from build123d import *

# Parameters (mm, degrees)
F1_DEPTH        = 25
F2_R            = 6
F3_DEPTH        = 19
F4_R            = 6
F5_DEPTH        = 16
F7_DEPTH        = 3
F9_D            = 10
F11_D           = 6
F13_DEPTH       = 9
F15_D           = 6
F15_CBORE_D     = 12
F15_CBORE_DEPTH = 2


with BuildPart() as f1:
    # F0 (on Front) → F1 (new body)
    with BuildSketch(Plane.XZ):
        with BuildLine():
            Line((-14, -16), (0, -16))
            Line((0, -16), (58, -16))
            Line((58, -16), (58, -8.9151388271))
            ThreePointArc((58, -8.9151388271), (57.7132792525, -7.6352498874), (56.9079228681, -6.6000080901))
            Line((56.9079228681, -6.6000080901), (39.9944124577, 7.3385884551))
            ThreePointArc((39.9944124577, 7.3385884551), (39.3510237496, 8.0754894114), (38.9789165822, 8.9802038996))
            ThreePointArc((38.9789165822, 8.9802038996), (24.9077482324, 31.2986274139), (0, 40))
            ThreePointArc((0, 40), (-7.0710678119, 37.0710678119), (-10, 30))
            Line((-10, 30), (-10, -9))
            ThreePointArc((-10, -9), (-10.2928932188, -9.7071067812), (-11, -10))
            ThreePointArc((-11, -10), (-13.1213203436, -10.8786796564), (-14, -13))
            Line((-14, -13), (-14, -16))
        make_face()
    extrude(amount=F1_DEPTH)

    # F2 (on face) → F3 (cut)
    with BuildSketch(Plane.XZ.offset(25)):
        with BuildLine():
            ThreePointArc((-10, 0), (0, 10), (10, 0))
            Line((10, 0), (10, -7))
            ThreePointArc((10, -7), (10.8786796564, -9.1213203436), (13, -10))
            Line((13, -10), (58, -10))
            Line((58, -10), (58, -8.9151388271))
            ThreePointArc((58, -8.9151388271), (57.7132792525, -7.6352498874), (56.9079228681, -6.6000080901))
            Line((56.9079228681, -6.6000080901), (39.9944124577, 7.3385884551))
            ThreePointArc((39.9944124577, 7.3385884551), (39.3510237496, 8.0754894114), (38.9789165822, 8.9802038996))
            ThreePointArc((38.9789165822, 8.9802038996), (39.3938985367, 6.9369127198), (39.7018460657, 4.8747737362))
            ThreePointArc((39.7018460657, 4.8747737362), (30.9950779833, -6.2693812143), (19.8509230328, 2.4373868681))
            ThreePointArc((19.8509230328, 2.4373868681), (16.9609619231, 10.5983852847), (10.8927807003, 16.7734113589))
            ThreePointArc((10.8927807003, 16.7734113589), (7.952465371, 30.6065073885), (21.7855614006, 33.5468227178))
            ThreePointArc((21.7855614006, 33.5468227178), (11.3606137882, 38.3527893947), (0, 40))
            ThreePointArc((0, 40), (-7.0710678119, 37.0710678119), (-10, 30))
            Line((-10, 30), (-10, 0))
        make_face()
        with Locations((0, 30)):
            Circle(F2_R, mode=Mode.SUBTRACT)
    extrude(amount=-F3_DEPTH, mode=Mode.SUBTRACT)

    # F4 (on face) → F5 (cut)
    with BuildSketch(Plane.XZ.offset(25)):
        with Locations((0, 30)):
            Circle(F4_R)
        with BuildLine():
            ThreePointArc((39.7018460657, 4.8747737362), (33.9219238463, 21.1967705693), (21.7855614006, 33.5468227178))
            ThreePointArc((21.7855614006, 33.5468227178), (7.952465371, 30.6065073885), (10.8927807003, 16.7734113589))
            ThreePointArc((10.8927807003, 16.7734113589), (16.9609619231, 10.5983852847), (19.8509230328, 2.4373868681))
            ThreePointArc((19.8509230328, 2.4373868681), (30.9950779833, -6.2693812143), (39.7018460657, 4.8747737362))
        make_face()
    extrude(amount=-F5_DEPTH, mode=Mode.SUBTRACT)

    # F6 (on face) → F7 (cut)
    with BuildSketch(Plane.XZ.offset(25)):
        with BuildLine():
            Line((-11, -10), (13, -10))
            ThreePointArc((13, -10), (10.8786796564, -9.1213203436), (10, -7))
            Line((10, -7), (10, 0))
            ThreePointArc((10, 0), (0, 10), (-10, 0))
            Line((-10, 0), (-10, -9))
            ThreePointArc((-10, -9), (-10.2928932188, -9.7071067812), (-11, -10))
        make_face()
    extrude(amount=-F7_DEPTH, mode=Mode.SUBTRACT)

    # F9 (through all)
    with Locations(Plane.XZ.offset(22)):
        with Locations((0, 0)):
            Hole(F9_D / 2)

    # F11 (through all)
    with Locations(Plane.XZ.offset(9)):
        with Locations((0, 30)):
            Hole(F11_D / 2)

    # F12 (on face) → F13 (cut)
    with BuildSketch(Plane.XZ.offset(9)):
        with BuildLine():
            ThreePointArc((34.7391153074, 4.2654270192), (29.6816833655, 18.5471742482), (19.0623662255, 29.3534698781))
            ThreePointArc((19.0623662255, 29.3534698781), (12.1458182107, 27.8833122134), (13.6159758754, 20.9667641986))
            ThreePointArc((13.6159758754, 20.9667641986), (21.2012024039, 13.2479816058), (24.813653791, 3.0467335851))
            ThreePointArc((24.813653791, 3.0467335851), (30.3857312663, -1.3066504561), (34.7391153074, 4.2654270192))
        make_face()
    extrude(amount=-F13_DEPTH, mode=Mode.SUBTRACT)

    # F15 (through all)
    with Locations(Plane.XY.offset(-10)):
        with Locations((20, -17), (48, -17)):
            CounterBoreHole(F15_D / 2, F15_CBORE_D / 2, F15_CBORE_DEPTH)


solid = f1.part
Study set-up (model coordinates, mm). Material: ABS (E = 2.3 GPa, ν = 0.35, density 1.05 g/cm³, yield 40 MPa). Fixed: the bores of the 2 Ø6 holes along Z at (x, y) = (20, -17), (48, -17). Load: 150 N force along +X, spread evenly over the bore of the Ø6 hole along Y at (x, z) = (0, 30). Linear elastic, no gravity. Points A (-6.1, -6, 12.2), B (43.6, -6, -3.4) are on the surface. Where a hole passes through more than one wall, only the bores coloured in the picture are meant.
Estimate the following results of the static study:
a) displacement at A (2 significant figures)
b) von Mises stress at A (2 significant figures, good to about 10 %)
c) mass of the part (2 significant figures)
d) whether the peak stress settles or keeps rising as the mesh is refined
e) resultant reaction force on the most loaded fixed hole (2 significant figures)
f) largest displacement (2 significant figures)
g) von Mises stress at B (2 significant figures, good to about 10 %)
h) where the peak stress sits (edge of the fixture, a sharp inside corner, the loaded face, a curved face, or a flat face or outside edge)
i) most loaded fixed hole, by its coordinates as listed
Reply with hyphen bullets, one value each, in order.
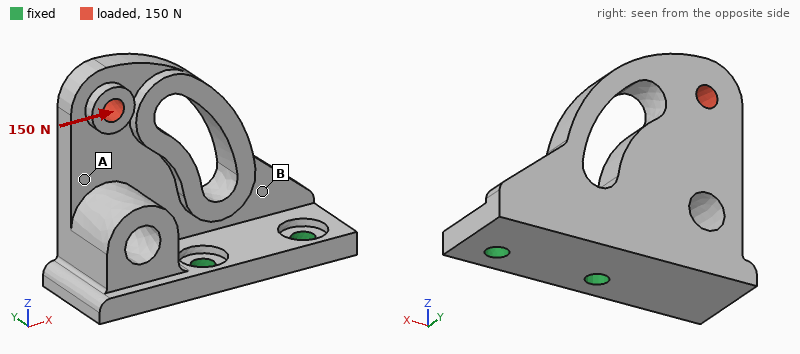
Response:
- 0.64 mm
- 2.5 MPa
- 29 g
- keeps rising
- 230 N
- 1.00 mm
- 7.3 MPa
- edge of the fixture
- (48, -17)
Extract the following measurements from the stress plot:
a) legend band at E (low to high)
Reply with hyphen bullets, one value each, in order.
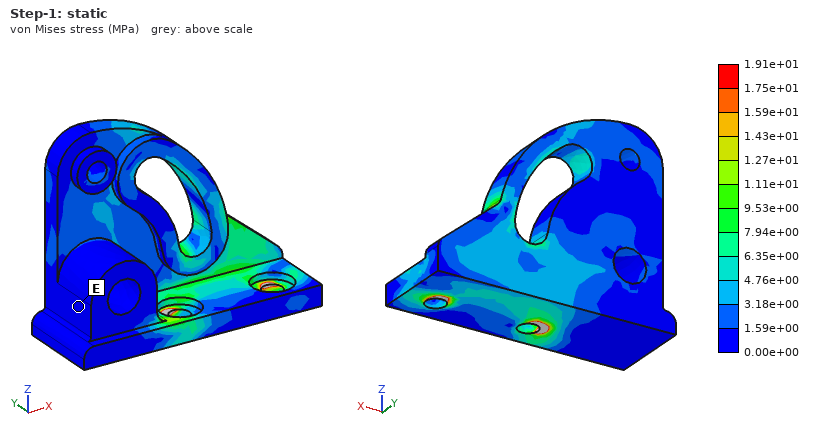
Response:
- 0.00e+00 to 1.59e+00 MPa
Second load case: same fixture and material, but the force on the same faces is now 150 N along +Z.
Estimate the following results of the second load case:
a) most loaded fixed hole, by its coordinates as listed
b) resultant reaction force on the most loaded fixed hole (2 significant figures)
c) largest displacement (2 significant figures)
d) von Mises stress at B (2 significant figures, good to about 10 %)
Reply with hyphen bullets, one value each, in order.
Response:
- (20, -17)
- 230 N
- 0.97 mm
- 4.1 MPa
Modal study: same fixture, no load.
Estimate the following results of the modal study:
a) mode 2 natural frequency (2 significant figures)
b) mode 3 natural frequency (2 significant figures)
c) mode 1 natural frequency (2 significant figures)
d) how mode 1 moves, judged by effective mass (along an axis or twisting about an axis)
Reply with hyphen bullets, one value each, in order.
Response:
- 840 Hz
- 1800 Hz
- 460 Hz
- along Y
